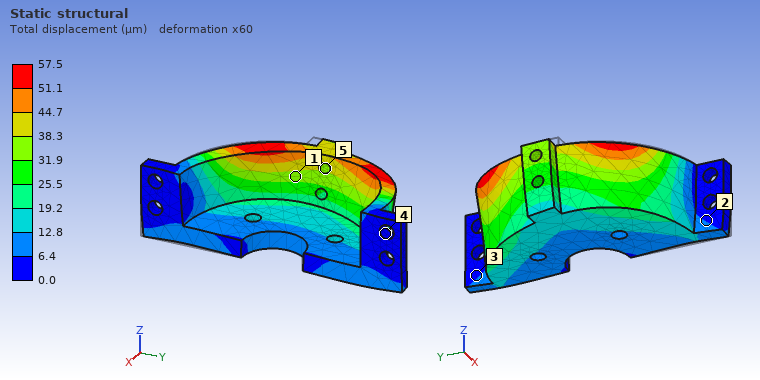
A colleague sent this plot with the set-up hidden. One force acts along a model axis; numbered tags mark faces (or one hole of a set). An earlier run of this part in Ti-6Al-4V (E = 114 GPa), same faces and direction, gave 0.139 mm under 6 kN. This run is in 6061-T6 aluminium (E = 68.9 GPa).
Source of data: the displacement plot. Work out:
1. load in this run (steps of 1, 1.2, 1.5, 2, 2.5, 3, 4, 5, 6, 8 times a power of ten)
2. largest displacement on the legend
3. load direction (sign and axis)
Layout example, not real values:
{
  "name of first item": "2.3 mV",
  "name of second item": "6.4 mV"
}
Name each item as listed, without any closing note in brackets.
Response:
{
  "load in this run": "1.5 kN",
  "largest displacement on the legend": "57.5 µm",
  "load direction": "+Y"
}
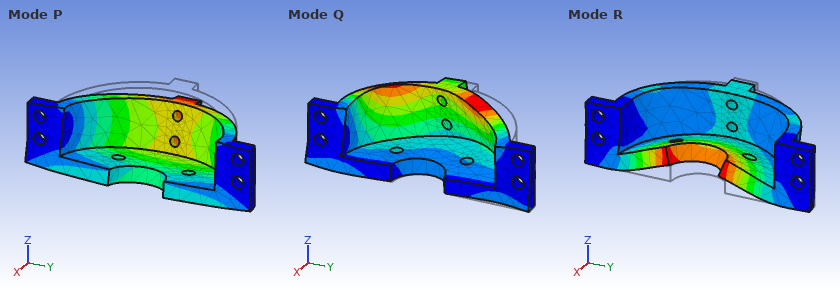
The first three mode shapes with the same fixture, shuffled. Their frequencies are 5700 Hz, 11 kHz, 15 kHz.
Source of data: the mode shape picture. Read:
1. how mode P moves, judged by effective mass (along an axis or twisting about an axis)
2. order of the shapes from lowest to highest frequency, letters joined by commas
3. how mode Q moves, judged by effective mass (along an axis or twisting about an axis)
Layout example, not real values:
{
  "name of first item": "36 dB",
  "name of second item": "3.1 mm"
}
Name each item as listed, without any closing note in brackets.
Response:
{
  "how mode P moves, judged by effective mass": "along Z",
  "order of the shapes from lowest to highest frequency, letters joined by commas": "P, Q, R",
  "how mode Q moves, judged by effective mass": "along Y"
}
